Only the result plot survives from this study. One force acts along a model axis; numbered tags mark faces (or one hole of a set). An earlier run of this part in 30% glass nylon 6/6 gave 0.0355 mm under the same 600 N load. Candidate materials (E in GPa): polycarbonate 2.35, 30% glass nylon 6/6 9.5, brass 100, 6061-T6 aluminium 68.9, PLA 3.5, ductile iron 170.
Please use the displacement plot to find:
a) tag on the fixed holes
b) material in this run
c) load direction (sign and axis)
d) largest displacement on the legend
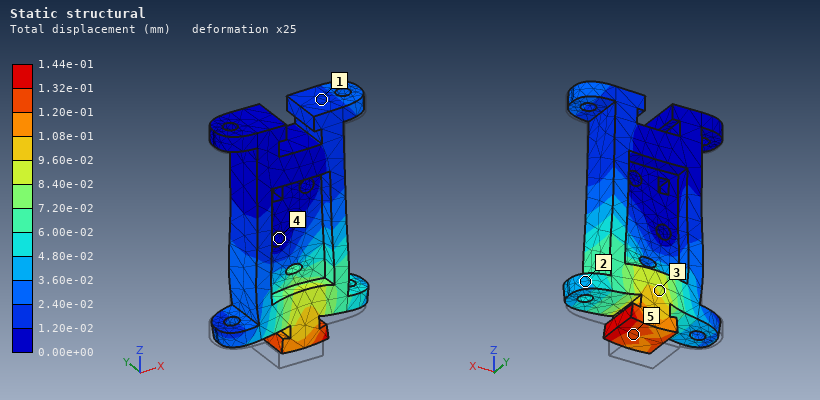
4
polycarbonate
+Z
1.44e-01 mm
